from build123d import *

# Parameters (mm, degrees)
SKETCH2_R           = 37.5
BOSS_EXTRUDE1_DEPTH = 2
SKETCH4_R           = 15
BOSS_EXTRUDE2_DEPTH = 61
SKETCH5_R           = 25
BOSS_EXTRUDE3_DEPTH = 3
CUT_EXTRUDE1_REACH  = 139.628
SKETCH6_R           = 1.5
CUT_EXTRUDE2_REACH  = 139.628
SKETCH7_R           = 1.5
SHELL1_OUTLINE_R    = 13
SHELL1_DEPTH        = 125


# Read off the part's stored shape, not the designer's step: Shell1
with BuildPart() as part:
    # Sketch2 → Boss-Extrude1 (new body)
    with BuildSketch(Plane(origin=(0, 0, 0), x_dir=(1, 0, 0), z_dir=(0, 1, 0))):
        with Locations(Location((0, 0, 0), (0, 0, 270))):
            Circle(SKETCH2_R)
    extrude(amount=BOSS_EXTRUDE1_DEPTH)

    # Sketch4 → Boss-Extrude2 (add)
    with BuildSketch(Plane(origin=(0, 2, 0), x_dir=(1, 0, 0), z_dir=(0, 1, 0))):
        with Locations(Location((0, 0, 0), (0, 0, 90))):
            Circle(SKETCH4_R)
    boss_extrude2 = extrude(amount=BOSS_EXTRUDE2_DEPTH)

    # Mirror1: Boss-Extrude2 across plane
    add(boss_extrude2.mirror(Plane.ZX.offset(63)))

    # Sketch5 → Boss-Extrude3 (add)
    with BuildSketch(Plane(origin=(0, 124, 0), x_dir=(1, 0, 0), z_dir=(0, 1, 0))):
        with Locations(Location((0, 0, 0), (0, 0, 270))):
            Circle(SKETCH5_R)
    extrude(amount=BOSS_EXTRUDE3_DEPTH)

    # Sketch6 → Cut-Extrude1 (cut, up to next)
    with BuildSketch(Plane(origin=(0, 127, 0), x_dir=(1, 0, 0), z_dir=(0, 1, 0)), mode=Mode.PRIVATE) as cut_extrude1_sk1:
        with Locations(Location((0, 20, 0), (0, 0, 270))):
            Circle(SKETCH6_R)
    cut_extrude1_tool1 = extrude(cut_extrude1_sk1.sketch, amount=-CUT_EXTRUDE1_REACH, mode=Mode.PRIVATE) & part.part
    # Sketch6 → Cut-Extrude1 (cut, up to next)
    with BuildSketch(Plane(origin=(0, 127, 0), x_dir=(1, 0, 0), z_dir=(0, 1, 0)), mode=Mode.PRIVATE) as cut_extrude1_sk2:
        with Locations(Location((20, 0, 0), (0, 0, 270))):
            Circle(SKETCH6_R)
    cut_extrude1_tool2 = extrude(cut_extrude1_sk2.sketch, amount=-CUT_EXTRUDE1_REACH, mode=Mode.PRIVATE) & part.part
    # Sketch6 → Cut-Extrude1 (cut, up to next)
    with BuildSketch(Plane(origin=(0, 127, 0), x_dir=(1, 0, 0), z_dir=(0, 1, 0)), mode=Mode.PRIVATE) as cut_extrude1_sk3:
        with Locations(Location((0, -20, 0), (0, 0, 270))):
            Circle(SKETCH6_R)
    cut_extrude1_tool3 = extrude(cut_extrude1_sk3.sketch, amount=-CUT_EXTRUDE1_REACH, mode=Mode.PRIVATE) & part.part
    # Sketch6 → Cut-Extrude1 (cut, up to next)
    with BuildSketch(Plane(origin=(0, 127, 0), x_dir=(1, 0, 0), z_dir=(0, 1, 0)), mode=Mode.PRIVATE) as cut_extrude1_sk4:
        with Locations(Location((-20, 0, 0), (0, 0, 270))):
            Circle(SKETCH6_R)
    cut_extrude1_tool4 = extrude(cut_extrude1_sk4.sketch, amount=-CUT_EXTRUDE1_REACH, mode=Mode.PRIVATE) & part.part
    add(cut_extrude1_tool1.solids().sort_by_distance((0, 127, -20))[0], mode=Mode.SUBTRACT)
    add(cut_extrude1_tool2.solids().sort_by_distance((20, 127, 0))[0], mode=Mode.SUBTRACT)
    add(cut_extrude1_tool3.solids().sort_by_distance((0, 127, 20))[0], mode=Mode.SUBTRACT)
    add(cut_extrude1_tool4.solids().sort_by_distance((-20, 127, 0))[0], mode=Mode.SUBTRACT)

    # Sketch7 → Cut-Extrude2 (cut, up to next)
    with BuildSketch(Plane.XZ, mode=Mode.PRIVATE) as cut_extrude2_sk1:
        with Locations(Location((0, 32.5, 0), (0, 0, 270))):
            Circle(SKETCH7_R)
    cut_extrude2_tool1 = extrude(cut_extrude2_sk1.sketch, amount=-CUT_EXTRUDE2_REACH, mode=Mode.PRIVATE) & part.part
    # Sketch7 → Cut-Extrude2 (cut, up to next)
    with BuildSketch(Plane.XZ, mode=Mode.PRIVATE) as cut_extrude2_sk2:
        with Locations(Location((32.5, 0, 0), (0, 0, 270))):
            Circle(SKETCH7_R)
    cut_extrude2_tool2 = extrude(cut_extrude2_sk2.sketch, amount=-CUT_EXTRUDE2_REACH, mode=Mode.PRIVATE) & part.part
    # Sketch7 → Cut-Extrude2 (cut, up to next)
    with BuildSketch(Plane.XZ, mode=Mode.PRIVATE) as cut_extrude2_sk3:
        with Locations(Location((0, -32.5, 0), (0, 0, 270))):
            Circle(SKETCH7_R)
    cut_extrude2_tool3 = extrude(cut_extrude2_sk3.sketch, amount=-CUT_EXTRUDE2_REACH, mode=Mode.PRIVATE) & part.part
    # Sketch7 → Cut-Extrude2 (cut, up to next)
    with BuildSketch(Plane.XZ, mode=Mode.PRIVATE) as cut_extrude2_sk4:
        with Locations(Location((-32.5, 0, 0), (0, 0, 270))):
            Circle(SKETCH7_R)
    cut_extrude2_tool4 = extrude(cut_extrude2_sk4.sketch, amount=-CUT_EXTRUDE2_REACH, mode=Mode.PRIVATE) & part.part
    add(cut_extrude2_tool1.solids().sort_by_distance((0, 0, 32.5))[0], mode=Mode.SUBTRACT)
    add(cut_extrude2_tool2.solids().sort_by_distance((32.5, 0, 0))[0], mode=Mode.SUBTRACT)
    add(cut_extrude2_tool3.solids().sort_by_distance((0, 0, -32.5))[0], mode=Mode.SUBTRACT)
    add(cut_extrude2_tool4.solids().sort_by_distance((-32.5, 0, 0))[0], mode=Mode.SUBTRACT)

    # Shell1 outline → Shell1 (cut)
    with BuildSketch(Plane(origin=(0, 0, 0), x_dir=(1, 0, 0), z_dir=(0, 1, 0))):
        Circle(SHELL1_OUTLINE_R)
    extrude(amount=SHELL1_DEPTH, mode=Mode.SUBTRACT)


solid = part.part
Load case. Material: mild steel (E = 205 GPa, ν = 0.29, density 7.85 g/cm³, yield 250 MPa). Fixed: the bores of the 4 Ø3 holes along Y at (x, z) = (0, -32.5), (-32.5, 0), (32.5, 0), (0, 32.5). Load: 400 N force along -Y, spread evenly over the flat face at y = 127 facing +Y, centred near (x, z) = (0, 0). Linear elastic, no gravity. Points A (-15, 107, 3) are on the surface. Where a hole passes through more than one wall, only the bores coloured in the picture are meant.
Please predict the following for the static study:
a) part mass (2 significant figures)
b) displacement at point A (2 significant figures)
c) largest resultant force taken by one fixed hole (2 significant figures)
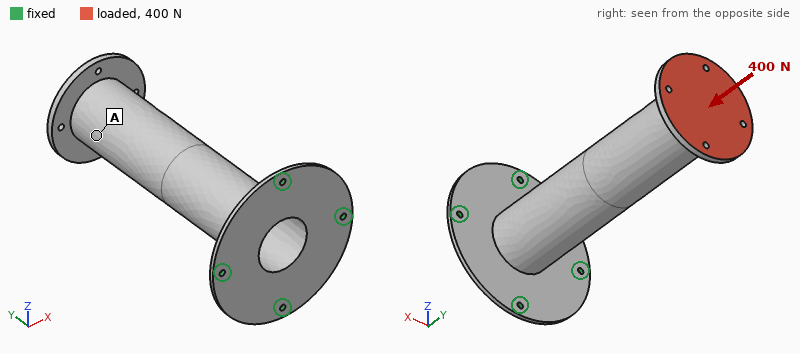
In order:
270 g
21 µm
120 N
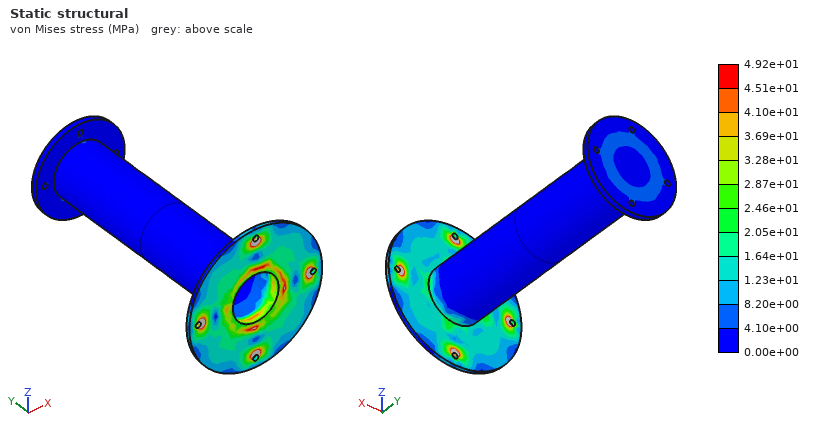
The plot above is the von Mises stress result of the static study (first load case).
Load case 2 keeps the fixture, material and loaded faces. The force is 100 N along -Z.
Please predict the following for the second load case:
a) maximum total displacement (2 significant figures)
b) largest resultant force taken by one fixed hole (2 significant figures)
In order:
0.27 mm
240 N
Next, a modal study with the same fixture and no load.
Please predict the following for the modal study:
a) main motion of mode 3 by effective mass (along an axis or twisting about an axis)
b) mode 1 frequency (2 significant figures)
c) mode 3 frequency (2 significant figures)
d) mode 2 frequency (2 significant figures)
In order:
along Y
320 Hz
1500 Hz
320 Hz
